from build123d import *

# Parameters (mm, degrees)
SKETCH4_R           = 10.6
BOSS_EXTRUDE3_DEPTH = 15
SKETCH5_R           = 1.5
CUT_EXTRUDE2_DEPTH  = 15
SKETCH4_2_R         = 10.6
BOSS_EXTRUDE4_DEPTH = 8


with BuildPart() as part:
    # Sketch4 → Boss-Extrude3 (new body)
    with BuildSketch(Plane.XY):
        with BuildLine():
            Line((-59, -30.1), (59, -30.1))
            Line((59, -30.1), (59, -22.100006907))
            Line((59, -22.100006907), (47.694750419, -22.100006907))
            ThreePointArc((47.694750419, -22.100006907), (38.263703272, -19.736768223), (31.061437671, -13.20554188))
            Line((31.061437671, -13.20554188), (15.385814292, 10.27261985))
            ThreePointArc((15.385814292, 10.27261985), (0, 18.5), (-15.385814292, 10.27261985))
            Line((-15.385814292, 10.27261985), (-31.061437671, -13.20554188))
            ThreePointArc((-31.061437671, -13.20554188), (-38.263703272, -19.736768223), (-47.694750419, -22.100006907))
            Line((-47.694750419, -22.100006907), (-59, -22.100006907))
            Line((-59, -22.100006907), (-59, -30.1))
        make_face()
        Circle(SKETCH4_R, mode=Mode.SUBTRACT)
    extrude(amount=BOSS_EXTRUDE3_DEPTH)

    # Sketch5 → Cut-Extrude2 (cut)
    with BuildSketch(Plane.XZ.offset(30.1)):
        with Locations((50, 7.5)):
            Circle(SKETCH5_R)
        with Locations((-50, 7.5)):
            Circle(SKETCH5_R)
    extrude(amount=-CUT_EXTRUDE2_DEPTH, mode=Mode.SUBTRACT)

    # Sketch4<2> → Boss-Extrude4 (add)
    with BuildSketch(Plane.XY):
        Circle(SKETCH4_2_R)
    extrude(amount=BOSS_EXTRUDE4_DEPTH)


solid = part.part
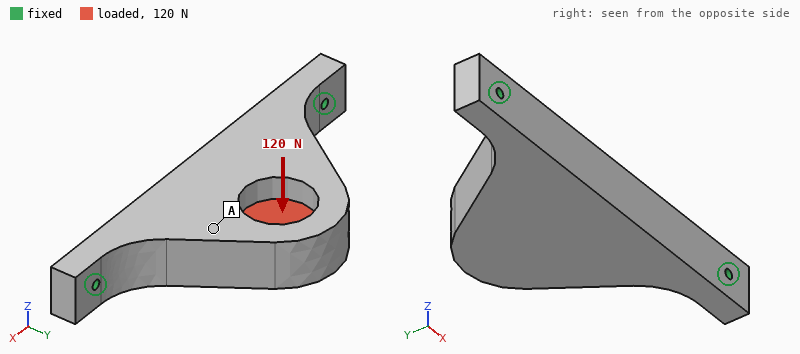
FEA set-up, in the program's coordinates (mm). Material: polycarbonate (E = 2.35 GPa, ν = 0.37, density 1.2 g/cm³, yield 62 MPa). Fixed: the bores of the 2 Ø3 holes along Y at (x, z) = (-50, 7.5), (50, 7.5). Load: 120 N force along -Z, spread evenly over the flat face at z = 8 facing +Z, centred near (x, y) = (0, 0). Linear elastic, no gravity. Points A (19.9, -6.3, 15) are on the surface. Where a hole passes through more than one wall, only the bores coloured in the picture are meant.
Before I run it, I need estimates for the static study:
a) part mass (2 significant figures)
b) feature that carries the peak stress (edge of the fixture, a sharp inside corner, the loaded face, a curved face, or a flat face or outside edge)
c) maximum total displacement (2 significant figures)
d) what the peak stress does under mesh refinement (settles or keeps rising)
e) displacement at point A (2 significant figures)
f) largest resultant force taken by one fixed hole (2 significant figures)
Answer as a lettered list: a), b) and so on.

a) 48 g
b) edge of the fixture
c) 0.84 mm
d) keeps rising
e) 0.41 mm
f) 60 N
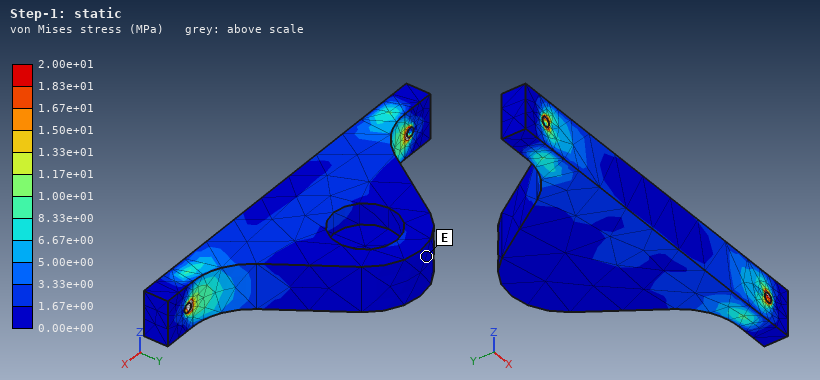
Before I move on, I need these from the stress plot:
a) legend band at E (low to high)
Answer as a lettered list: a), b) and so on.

a) 0.00e+00 to 1.67e+00 MPa
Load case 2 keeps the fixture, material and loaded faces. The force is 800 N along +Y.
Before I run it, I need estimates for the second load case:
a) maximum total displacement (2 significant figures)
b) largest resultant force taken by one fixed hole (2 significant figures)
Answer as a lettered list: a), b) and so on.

a) 0.27 mm
b) 560 N
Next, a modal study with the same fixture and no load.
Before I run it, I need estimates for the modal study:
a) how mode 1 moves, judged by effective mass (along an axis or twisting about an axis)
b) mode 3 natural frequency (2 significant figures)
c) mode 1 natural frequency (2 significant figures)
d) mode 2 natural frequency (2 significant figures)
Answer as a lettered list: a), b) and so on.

a) along Z
b) 1500 Hz
c) 500 Hz
d) 1400 Hz
